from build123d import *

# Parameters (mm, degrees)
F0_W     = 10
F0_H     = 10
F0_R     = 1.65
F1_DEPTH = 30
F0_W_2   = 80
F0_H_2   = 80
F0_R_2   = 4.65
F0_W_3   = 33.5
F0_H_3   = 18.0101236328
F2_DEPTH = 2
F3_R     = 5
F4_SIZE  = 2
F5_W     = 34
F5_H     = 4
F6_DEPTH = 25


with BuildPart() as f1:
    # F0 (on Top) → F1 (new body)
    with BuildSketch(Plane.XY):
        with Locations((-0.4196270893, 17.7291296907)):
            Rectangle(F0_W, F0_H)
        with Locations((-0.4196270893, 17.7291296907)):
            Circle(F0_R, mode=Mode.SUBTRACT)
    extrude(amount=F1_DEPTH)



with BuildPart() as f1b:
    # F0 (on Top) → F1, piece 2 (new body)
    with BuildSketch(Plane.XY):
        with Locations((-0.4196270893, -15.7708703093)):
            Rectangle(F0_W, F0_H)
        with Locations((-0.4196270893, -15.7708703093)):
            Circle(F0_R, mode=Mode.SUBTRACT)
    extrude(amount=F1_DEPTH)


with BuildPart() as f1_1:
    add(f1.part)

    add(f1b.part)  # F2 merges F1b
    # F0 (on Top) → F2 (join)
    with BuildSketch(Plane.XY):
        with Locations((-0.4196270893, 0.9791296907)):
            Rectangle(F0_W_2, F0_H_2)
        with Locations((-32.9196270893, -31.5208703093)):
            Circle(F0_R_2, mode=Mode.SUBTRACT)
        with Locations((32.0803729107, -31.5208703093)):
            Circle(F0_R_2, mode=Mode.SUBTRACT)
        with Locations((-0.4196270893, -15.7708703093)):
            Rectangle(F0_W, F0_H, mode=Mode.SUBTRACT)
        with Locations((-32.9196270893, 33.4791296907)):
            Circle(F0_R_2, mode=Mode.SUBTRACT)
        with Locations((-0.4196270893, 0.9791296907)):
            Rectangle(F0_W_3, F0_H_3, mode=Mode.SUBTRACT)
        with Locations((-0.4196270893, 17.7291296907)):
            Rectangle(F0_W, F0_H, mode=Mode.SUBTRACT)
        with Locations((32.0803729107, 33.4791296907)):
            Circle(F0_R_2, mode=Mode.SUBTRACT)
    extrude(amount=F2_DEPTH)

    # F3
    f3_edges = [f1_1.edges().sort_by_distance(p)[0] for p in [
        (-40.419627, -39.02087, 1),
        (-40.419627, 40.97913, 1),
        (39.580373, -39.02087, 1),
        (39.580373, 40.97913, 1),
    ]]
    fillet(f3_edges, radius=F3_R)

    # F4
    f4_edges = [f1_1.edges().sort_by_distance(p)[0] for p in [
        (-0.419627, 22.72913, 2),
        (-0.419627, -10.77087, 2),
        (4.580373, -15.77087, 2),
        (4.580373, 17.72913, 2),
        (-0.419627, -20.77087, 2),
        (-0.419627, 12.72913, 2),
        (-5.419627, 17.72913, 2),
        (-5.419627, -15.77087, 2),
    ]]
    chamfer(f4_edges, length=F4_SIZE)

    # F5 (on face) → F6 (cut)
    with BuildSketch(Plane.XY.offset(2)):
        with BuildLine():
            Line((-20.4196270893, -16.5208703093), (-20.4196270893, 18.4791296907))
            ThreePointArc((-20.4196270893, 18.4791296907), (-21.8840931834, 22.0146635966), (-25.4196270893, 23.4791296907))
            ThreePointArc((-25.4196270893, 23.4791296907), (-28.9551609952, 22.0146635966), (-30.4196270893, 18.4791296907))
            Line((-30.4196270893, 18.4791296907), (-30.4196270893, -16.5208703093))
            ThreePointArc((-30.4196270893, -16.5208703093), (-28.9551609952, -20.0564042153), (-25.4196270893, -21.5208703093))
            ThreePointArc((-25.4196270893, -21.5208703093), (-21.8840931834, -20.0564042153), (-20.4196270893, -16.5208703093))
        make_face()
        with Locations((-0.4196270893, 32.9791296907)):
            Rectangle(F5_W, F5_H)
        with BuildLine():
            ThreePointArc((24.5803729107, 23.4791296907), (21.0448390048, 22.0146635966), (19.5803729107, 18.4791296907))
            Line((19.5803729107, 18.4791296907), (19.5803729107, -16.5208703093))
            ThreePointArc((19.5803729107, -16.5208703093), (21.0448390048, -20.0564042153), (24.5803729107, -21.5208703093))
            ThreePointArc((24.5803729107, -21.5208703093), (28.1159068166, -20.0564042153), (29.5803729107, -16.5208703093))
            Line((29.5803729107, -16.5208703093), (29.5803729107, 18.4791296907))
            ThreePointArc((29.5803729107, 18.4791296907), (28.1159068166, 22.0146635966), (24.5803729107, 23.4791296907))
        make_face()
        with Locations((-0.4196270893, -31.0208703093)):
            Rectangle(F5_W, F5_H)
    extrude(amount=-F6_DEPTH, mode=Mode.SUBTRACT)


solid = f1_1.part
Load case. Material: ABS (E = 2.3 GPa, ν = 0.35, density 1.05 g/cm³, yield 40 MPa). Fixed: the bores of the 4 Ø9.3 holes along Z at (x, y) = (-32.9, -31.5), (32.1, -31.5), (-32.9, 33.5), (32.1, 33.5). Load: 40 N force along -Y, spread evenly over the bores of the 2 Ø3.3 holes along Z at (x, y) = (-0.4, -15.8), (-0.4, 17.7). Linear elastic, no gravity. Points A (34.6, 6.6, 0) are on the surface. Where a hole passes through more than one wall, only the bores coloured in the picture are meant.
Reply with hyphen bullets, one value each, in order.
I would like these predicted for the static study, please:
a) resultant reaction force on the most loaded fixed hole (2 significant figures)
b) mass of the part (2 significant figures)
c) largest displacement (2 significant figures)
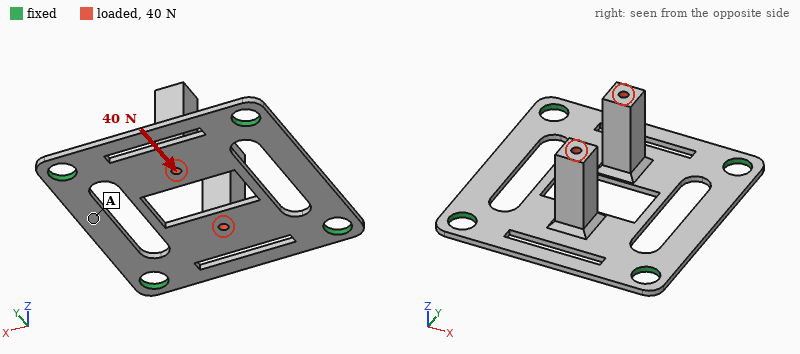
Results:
- 13 N
- 15 g
- 1.2 mm
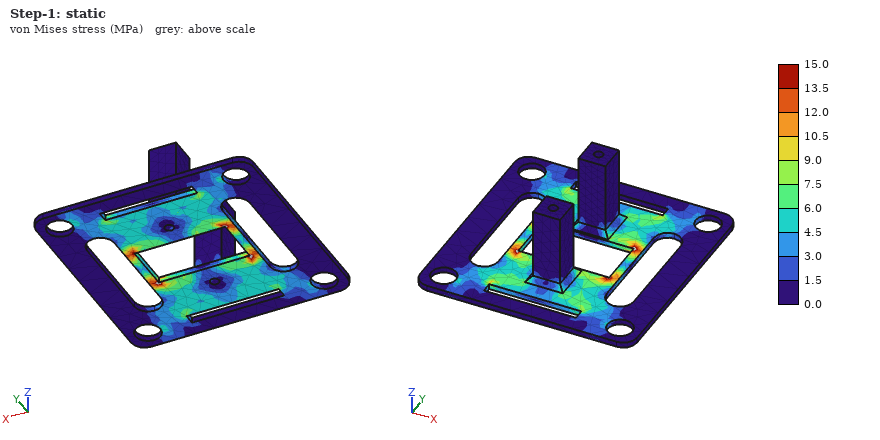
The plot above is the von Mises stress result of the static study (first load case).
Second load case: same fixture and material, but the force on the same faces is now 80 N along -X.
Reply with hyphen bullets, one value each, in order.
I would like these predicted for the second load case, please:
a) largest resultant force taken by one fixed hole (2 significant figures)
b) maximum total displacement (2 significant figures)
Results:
- 26 N
- 1.2 mm
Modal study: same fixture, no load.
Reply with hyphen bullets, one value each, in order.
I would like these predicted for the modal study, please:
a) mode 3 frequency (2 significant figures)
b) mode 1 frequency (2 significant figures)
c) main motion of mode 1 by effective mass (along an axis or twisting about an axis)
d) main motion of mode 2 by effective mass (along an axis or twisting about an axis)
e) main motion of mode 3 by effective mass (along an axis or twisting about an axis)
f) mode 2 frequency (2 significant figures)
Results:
- 570 Hz
- 260 Hz
- along Z
- along Y
- along Z
- 430 Hz
